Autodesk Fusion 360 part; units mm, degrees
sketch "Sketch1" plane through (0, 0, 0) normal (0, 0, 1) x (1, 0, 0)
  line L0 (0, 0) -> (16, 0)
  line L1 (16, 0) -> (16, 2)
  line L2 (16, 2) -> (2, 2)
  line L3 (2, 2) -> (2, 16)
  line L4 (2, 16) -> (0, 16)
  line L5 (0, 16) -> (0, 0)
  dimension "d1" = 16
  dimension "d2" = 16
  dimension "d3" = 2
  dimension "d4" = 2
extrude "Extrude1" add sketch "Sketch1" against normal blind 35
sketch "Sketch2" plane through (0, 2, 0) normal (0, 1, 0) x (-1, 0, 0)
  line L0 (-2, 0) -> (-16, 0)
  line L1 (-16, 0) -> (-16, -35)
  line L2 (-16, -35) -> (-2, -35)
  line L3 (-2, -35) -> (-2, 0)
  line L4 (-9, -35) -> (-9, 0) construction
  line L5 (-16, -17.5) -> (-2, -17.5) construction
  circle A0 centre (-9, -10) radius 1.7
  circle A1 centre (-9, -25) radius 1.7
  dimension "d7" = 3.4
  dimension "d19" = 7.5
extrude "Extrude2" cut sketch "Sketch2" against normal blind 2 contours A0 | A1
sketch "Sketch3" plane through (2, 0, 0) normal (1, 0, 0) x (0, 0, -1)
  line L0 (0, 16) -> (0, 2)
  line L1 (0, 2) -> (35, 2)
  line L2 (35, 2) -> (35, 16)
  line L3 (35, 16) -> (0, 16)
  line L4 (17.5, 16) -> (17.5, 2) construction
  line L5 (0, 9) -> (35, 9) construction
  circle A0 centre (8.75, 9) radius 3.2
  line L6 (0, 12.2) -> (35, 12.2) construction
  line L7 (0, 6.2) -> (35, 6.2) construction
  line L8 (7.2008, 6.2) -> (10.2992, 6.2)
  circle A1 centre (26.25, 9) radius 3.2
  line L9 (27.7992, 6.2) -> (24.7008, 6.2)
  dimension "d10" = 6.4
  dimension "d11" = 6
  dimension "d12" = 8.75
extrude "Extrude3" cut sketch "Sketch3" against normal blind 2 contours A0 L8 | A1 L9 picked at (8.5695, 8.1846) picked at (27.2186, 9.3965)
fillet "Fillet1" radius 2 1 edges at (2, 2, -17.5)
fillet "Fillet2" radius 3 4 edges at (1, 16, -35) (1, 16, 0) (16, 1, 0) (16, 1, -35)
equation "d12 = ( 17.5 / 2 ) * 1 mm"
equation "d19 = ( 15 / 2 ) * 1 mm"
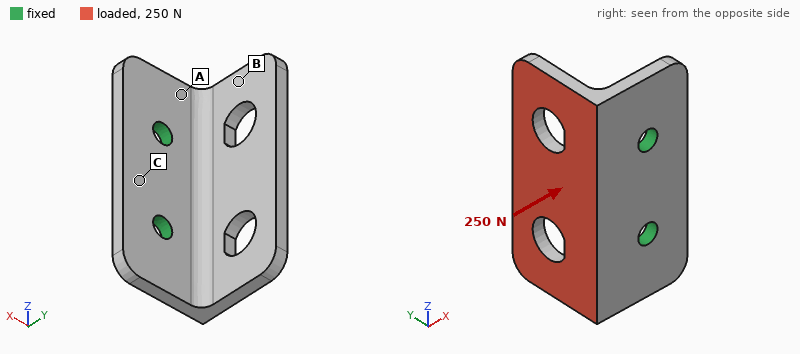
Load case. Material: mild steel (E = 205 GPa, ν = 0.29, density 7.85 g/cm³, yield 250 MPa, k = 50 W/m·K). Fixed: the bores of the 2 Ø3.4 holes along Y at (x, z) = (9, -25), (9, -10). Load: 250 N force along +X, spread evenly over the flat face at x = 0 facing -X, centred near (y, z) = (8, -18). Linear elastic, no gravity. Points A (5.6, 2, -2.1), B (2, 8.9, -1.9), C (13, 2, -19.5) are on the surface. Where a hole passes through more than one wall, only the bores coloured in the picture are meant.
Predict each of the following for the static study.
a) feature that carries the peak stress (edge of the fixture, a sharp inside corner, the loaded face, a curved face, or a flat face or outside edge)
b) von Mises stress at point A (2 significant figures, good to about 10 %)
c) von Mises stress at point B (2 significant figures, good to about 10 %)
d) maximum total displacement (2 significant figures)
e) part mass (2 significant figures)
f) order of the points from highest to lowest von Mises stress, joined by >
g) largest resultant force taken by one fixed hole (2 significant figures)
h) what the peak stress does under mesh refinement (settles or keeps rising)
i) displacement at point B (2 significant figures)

edge of the fixture
55 MPa
25 MPa
53 µm
15 g
A > B > C
130 N
keeps rising
24 µm
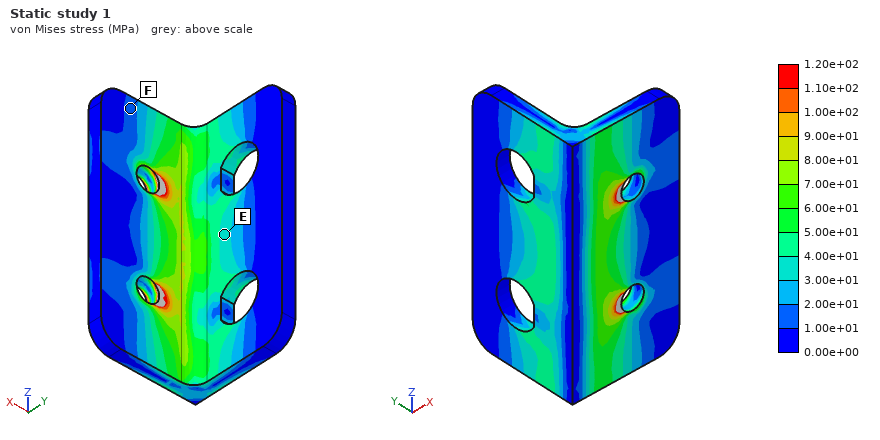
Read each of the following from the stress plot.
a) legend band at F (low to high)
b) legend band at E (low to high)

1.00e+01 to 2.00e+01 MPa
3.00e+01 to 4.00e+01 MPa
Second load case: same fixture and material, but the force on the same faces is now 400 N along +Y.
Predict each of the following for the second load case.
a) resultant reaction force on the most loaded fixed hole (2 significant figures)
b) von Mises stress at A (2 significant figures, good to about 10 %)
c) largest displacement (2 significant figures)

200 N
59 MPa
54 µm
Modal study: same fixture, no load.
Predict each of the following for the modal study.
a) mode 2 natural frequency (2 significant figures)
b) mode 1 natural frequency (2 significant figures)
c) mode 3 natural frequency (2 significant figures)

6900 Hz
4500 Hz
11 kHz
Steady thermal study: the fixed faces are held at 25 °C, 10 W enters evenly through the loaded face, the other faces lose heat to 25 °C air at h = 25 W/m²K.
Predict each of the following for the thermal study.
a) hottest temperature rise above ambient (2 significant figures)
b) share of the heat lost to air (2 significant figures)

43 K
8.2 %
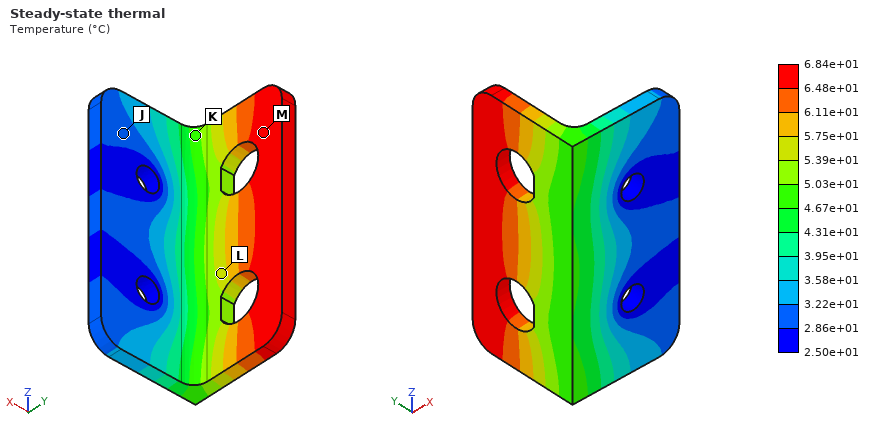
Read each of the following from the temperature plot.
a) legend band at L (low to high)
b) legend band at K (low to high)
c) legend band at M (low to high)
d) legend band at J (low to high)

5.39e+01 to 5.75e+01 °C
4.67e+01 to 5.03e+01 °C
6.48e+01 to 6.84e+01 °C
2.86e+01 to 3.22e+01 °C
